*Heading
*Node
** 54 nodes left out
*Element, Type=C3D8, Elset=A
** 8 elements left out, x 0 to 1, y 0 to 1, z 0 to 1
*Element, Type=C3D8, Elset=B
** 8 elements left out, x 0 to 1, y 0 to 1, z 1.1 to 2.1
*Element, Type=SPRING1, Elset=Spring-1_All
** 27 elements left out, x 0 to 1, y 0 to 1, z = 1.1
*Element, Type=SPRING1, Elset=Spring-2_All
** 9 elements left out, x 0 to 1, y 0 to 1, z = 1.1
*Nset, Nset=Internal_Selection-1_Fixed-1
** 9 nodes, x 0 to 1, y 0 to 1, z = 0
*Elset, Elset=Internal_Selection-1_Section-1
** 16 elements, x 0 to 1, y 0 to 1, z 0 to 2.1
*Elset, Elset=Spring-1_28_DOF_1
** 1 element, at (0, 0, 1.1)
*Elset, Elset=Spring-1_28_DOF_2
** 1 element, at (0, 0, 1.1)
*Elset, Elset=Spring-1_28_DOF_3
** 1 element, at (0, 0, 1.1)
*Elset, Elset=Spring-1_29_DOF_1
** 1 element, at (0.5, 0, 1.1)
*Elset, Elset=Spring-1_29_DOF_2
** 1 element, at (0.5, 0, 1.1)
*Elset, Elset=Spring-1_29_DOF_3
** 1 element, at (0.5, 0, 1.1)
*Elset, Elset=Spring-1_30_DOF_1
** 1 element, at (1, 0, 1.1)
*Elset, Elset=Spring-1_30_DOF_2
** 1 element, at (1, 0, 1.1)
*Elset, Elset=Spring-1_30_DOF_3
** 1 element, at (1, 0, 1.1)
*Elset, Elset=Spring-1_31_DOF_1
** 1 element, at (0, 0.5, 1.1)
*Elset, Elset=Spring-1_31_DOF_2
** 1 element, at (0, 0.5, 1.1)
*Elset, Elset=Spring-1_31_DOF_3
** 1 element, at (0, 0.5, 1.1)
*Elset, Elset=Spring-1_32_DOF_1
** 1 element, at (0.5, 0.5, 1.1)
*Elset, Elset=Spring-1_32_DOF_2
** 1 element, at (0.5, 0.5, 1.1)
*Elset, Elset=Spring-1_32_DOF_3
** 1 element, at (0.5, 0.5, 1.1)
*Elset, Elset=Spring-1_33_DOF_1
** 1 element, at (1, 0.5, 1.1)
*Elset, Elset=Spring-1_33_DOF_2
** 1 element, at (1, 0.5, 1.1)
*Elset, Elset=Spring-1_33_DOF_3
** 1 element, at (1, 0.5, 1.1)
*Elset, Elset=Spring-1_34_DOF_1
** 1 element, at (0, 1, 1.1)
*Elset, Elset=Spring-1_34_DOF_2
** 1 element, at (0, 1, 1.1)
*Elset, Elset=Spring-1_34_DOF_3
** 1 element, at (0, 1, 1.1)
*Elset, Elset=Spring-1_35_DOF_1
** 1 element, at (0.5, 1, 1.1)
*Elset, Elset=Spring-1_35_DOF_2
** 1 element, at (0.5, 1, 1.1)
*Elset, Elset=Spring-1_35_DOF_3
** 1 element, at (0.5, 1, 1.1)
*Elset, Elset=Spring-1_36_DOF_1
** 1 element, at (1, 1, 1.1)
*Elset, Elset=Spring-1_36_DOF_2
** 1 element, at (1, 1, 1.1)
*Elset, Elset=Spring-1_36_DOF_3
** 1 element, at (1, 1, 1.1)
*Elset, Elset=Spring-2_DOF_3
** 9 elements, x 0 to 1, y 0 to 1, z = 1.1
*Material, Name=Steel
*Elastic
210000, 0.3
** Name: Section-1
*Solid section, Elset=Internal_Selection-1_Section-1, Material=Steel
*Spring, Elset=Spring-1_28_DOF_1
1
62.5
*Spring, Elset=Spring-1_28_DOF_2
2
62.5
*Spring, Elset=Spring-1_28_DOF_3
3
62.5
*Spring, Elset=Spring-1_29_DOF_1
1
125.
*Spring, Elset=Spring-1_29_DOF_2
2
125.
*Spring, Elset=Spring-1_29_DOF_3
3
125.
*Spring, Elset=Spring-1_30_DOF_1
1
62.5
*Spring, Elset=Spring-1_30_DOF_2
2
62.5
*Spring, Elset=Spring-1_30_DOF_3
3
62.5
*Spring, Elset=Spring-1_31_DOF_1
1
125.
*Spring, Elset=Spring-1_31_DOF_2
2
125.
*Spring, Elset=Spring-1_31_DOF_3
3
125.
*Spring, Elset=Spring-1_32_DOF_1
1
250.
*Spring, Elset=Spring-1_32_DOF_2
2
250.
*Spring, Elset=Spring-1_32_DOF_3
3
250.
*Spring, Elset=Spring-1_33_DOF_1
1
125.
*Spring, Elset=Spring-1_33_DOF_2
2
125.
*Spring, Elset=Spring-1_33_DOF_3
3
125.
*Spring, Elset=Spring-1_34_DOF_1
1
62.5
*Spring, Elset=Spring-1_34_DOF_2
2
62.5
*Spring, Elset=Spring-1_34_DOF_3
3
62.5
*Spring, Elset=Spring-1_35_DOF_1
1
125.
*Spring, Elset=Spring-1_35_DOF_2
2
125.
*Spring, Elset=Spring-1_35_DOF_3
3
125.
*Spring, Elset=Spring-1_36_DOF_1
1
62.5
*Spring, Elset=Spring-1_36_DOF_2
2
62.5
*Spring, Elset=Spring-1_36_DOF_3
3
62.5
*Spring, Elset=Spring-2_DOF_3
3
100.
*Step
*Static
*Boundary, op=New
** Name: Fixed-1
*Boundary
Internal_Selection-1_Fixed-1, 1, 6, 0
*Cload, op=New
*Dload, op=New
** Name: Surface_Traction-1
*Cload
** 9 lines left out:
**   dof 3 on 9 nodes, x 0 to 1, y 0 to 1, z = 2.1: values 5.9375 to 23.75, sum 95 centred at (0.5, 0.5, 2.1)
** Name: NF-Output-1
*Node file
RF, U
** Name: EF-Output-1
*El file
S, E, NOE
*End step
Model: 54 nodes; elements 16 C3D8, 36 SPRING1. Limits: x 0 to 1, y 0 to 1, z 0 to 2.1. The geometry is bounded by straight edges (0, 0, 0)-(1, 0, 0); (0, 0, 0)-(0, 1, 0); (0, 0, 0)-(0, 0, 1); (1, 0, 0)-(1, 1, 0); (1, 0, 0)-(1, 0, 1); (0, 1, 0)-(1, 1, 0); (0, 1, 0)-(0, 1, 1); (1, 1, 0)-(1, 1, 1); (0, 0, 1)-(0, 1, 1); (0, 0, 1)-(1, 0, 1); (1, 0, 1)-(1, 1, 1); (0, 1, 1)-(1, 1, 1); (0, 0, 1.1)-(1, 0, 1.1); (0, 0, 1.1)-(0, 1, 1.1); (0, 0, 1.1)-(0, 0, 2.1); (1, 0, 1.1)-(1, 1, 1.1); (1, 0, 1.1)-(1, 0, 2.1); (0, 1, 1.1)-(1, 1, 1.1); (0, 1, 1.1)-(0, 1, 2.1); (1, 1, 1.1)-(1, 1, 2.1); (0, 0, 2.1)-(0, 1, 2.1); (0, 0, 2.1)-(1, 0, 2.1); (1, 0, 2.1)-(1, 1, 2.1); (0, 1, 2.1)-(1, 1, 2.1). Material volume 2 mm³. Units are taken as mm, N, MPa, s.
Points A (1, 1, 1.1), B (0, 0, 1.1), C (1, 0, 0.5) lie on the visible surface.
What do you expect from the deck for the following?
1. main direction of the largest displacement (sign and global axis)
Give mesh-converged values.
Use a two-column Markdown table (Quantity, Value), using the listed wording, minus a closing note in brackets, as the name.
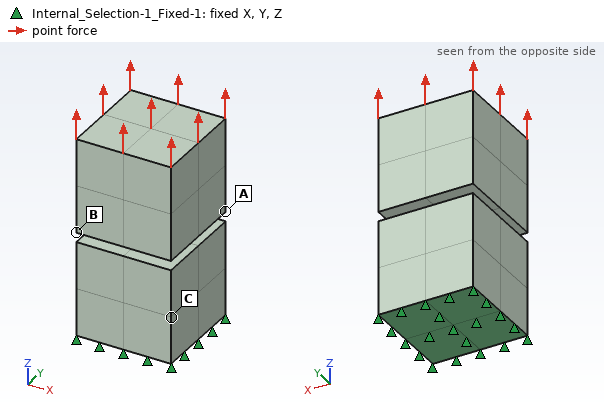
| Quantity | Value |
|---|---|
| main direction of the largest displacement | +Z |
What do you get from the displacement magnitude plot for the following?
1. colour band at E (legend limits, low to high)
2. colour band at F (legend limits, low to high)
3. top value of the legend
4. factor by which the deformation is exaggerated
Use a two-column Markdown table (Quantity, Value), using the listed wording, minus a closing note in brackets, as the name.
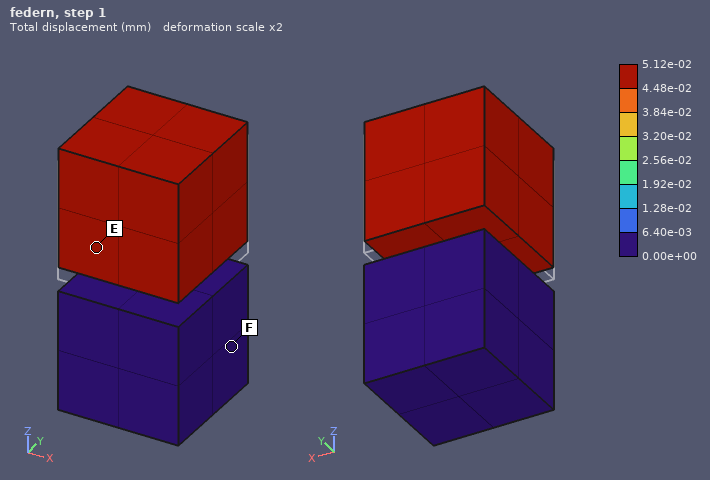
| Quantity | Value |
|---|---|
| colour band at E | 4.48e-02 to 5.12e-02 mm |
| colour band at F | 0.00e+00 to 6.40e-03 mm |
| top value of the legend | 5.12e-02 mm |
| factor by which the deformation is exaggerated | 2 |
